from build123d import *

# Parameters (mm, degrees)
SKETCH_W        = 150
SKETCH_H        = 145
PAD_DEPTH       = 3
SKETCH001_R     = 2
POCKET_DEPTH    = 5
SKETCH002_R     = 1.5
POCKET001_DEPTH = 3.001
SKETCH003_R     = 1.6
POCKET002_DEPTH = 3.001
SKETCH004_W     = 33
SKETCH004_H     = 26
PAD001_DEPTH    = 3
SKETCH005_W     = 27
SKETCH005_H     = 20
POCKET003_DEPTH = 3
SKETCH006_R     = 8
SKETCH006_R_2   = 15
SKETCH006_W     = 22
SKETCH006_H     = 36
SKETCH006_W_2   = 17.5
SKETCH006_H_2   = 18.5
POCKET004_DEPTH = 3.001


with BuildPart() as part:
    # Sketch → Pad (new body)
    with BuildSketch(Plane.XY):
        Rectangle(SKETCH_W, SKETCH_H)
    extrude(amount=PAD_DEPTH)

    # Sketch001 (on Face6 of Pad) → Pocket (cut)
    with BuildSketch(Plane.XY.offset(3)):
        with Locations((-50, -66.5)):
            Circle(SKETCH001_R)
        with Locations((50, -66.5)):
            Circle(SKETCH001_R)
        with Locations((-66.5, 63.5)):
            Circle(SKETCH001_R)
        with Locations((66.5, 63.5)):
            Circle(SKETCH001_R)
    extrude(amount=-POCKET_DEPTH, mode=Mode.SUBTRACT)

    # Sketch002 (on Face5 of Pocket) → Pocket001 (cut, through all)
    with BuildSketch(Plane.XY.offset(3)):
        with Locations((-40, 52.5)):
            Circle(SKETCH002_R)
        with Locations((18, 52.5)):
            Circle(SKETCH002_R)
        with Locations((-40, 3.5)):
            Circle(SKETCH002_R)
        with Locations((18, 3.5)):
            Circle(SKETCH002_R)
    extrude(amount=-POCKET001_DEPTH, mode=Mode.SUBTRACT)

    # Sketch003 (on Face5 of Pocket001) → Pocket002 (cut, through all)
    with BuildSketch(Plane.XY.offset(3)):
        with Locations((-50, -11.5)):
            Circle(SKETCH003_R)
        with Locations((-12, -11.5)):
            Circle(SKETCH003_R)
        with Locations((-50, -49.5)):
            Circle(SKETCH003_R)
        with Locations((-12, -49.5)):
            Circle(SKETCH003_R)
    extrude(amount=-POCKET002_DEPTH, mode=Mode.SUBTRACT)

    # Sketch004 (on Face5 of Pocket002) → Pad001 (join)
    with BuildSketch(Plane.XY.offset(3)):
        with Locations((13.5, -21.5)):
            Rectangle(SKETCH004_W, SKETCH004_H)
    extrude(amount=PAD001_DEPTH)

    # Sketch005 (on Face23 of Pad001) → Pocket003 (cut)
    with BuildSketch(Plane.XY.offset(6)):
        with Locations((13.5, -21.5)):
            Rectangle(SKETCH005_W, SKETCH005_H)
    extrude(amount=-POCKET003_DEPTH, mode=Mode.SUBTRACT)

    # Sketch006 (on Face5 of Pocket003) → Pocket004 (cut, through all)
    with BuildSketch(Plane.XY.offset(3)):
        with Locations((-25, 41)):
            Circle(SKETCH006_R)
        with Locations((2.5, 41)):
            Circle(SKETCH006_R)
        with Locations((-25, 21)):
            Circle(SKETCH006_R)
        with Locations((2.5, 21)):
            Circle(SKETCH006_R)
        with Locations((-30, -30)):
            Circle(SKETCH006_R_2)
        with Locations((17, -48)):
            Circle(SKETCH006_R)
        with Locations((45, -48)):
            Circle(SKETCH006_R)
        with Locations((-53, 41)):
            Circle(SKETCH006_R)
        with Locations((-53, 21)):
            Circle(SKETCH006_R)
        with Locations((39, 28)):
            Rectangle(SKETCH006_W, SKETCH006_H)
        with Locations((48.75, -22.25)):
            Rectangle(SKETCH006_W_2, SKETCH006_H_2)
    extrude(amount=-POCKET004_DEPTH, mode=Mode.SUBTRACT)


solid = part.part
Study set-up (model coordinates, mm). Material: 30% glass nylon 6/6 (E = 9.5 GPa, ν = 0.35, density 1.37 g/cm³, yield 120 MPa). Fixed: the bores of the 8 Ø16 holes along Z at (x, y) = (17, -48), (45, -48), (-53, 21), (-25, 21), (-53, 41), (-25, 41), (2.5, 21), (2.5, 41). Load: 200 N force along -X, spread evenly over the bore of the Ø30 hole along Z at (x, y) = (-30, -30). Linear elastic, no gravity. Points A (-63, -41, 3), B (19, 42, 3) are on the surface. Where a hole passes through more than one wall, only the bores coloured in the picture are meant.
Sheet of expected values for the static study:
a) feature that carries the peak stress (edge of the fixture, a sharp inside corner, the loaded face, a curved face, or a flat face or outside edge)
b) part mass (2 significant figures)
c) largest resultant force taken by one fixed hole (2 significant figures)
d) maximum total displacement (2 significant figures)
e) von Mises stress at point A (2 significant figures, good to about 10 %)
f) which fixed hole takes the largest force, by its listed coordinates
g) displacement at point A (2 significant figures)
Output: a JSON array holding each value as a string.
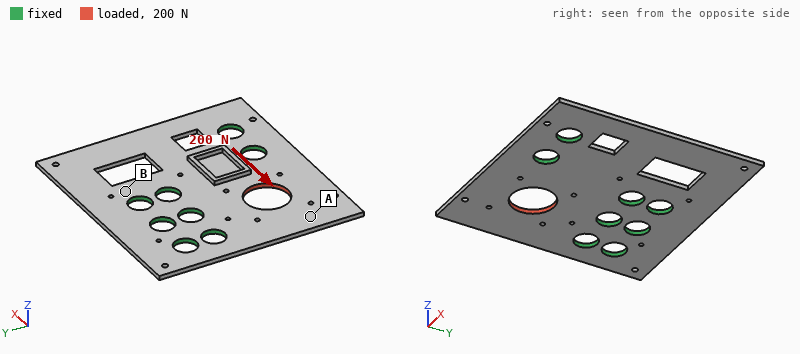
["a curved face", "76 g", "100 N", "6.8 µm", "0.39 MPa", "(17, -48)", "5.8 µm"]
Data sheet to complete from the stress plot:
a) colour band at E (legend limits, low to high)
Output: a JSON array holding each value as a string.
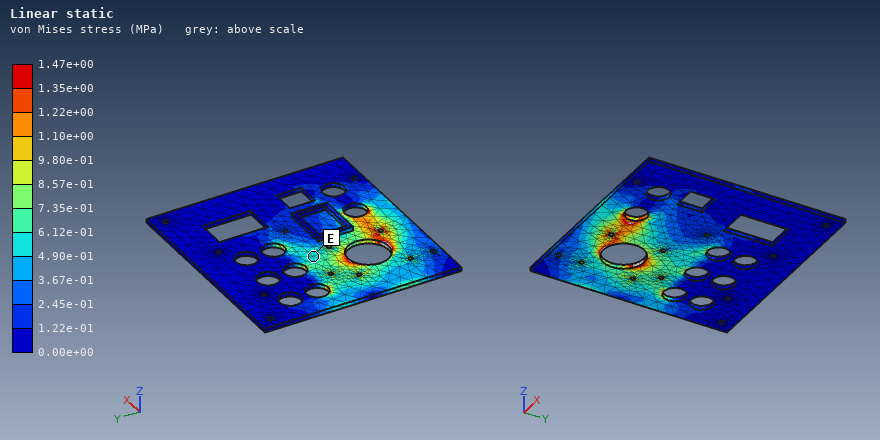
["4.90e-01 to 6.12e-01 MPa"]
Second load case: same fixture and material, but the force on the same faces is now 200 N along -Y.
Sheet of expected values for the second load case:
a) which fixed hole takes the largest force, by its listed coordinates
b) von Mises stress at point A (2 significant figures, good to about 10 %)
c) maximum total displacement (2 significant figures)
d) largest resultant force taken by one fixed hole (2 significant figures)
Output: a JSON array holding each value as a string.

["(-53, 21)", "0.30 MPa", "7.0 µm", "71 N"]
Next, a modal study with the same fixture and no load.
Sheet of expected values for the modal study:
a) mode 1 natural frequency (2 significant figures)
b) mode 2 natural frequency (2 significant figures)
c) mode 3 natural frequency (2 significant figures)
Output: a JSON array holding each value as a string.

["320 Hz", "320 Hz", "740 Hz"]
